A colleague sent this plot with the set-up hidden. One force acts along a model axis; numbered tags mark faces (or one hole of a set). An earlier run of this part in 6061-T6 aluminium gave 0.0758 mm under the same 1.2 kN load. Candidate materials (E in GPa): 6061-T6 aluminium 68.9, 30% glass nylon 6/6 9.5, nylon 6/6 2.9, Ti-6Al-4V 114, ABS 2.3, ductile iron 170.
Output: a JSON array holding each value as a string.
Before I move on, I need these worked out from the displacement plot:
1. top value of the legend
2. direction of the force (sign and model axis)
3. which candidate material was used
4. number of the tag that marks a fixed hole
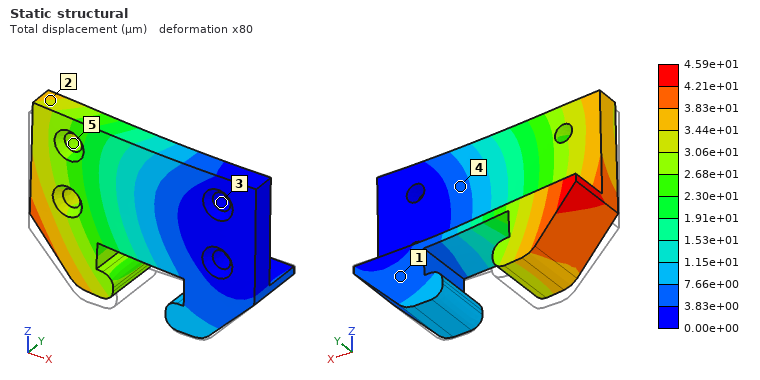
["4.59e+01 µm", "+Z", "Ti-6Al-4V", "3"]
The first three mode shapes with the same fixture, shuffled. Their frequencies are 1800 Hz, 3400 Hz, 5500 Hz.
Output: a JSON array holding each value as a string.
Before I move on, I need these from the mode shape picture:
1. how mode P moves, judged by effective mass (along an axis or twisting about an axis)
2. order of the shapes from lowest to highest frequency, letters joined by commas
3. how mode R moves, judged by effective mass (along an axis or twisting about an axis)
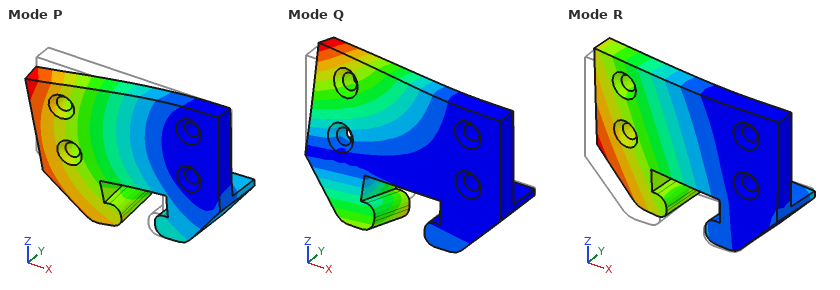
["along Z", "R, Q, P", "along Y"]
